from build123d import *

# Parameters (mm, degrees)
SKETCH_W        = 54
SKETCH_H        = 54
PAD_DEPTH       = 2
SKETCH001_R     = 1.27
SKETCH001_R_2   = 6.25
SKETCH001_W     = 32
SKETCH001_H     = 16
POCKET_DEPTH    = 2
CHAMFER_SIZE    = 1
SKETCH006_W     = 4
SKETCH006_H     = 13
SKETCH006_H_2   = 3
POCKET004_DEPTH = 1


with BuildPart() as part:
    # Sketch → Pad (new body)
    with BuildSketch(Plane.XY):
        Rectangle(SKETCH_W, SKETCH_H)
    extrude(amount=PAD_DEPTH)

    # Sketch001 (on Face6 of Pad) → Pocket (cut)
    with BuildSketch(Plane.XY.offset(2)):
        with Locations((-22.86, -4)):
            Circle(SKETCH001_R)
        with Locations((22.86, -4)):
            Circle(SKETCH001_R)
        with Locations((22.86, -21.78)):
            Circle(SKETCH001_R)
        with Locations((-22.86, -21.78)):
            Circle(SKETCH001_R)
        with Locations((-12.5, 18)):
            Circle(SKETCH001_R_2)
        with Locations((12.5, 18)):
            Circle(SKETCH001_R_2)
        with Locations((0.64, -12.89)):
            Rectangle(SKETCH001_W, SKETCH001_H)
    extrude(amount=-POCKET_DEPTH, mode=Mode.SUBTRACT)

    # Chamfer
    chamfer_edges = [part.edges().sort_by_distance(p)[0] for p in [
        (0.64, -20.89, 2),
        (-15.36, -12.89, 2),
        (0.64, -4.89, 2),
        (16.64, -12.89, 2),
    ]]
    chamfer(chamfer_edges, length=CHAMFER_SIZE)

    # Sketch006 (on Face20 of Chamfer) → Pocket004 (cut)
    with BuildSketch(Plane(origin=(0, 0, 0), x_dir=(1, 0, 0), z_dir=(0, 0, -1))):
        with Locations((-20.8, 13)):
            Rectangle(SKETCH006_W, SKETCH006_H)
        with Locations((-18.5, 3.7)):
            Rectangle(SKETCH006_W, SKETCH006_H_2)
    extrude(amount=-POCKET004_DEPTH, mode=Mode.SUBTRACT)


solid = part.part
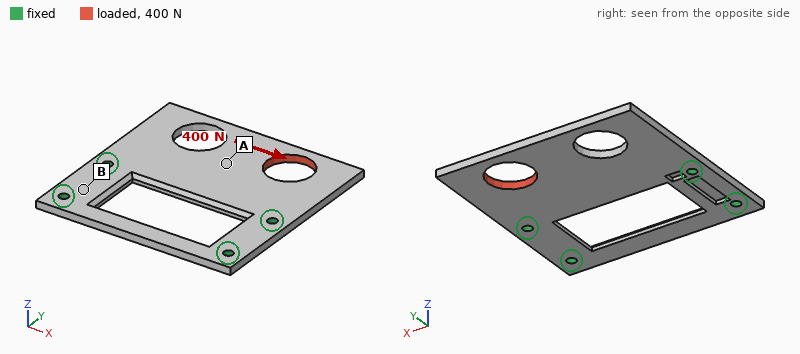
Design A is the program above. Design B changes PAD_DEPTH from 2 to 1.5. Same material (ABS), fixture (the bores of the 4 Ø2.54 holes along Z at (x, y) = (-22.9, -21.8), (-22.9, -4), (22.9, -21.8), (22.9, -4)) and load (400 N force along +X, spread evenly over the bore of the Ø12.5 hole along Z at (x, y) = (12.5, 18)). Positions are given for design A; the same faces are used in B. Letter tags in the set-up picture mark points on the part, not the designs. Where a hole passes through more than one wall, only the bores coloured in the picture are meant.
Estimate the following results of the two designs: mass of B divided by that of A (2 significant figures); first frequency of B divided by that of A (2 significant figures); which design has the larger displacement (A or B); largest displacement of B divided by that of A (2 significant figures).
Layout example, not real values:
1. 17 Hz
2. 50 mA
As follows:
1. 0.74
2. 0.76
3. B
4. 1.4
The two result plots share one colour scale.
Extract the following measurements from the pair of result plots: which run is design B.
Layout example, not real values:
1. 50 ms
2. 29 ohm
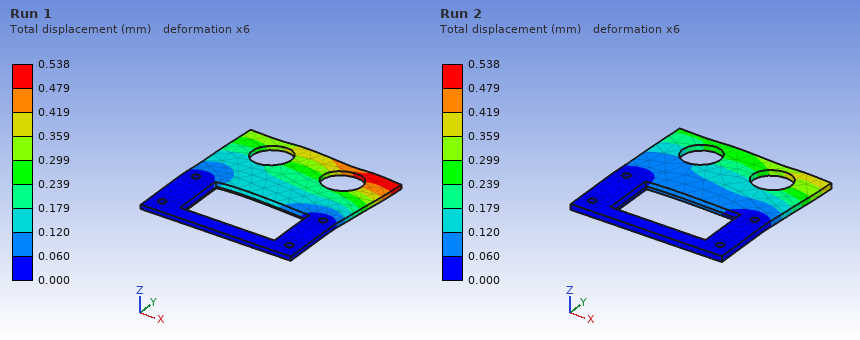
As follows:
1. Run 1
